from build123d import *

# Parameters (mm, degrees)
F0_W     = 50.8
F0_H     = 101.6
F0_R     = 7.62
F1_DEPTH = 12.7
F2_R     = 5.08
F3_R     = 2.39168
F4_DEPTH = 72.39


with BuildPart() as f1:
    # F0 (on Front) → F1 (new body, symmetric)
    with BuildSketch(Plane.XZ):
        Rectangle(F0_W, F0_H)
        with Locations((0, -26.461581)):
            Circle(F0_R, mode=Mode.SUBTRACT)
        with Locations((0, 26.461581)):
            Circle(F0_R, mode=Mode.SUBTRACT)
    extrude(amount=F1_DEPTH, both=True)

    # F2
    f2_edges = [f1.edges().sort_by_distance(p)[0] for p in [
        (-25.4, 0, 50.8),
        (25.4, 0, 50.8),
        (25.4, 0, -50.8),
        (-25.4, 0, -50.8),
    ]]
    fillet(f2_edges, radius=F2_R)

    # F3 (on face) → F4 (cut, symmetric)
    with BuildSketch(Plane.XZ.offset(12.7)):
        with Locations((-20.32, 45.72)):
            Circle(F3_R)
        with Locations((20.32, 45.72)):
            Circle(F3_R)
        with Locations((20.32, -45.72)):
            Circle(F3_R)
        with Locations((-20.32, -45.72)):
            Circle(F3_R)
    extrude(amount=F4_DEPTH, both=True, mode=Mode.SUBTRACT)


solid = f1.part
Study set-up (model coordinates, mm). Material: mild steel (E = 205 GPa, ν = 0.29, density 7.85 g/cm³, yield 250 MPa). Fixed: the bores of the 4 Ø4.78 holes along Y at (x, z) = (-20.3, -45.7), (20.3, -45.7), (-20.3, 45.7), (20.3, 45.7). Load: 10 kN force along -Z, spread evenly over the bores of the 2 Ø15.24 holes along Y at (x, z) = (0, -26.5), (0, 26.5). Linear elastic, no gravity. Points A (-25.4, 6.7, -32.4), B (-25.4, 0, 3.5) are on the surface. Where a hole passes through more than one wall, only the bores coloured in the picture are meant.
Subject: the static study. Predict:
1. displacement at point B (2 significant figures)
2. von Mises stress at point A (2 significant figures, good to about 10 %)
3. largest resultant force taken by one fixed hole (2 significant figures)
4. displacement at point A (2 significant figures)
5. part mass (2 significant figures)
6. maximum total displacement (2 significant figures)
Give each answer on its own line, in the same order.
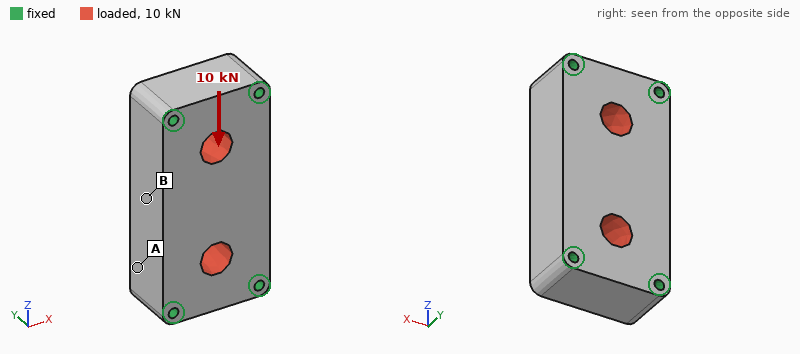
0.67 µm
4.7 MPa
2.6 kN
0.31 µm
940 g
0.94 µm
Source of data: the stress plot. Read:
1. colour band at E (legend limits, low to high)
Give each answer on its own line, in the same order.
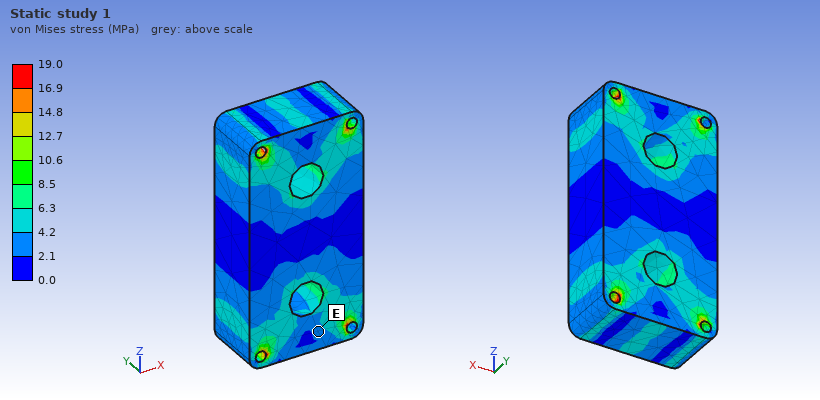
2.1 to 4.2 MPa
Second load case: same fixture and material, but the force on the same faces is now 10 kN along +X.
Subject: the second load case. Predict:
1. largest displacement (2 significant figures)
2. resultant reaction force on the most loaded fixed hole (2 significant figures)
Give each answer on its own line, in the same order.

2.2 µm
3.1 kN
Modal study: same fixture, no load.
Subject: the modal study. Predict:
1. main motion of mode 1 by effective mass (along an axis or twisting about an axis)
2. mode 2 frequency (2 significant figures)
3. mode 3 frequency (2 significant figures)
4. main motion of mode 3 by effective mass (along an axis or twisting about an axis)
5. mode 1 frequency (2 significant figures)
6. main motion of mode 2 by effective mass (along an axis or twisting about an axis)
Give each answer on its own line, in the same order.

along Y
12 kHz
13 kHz
twisting about Z
9600 Hz
along X
